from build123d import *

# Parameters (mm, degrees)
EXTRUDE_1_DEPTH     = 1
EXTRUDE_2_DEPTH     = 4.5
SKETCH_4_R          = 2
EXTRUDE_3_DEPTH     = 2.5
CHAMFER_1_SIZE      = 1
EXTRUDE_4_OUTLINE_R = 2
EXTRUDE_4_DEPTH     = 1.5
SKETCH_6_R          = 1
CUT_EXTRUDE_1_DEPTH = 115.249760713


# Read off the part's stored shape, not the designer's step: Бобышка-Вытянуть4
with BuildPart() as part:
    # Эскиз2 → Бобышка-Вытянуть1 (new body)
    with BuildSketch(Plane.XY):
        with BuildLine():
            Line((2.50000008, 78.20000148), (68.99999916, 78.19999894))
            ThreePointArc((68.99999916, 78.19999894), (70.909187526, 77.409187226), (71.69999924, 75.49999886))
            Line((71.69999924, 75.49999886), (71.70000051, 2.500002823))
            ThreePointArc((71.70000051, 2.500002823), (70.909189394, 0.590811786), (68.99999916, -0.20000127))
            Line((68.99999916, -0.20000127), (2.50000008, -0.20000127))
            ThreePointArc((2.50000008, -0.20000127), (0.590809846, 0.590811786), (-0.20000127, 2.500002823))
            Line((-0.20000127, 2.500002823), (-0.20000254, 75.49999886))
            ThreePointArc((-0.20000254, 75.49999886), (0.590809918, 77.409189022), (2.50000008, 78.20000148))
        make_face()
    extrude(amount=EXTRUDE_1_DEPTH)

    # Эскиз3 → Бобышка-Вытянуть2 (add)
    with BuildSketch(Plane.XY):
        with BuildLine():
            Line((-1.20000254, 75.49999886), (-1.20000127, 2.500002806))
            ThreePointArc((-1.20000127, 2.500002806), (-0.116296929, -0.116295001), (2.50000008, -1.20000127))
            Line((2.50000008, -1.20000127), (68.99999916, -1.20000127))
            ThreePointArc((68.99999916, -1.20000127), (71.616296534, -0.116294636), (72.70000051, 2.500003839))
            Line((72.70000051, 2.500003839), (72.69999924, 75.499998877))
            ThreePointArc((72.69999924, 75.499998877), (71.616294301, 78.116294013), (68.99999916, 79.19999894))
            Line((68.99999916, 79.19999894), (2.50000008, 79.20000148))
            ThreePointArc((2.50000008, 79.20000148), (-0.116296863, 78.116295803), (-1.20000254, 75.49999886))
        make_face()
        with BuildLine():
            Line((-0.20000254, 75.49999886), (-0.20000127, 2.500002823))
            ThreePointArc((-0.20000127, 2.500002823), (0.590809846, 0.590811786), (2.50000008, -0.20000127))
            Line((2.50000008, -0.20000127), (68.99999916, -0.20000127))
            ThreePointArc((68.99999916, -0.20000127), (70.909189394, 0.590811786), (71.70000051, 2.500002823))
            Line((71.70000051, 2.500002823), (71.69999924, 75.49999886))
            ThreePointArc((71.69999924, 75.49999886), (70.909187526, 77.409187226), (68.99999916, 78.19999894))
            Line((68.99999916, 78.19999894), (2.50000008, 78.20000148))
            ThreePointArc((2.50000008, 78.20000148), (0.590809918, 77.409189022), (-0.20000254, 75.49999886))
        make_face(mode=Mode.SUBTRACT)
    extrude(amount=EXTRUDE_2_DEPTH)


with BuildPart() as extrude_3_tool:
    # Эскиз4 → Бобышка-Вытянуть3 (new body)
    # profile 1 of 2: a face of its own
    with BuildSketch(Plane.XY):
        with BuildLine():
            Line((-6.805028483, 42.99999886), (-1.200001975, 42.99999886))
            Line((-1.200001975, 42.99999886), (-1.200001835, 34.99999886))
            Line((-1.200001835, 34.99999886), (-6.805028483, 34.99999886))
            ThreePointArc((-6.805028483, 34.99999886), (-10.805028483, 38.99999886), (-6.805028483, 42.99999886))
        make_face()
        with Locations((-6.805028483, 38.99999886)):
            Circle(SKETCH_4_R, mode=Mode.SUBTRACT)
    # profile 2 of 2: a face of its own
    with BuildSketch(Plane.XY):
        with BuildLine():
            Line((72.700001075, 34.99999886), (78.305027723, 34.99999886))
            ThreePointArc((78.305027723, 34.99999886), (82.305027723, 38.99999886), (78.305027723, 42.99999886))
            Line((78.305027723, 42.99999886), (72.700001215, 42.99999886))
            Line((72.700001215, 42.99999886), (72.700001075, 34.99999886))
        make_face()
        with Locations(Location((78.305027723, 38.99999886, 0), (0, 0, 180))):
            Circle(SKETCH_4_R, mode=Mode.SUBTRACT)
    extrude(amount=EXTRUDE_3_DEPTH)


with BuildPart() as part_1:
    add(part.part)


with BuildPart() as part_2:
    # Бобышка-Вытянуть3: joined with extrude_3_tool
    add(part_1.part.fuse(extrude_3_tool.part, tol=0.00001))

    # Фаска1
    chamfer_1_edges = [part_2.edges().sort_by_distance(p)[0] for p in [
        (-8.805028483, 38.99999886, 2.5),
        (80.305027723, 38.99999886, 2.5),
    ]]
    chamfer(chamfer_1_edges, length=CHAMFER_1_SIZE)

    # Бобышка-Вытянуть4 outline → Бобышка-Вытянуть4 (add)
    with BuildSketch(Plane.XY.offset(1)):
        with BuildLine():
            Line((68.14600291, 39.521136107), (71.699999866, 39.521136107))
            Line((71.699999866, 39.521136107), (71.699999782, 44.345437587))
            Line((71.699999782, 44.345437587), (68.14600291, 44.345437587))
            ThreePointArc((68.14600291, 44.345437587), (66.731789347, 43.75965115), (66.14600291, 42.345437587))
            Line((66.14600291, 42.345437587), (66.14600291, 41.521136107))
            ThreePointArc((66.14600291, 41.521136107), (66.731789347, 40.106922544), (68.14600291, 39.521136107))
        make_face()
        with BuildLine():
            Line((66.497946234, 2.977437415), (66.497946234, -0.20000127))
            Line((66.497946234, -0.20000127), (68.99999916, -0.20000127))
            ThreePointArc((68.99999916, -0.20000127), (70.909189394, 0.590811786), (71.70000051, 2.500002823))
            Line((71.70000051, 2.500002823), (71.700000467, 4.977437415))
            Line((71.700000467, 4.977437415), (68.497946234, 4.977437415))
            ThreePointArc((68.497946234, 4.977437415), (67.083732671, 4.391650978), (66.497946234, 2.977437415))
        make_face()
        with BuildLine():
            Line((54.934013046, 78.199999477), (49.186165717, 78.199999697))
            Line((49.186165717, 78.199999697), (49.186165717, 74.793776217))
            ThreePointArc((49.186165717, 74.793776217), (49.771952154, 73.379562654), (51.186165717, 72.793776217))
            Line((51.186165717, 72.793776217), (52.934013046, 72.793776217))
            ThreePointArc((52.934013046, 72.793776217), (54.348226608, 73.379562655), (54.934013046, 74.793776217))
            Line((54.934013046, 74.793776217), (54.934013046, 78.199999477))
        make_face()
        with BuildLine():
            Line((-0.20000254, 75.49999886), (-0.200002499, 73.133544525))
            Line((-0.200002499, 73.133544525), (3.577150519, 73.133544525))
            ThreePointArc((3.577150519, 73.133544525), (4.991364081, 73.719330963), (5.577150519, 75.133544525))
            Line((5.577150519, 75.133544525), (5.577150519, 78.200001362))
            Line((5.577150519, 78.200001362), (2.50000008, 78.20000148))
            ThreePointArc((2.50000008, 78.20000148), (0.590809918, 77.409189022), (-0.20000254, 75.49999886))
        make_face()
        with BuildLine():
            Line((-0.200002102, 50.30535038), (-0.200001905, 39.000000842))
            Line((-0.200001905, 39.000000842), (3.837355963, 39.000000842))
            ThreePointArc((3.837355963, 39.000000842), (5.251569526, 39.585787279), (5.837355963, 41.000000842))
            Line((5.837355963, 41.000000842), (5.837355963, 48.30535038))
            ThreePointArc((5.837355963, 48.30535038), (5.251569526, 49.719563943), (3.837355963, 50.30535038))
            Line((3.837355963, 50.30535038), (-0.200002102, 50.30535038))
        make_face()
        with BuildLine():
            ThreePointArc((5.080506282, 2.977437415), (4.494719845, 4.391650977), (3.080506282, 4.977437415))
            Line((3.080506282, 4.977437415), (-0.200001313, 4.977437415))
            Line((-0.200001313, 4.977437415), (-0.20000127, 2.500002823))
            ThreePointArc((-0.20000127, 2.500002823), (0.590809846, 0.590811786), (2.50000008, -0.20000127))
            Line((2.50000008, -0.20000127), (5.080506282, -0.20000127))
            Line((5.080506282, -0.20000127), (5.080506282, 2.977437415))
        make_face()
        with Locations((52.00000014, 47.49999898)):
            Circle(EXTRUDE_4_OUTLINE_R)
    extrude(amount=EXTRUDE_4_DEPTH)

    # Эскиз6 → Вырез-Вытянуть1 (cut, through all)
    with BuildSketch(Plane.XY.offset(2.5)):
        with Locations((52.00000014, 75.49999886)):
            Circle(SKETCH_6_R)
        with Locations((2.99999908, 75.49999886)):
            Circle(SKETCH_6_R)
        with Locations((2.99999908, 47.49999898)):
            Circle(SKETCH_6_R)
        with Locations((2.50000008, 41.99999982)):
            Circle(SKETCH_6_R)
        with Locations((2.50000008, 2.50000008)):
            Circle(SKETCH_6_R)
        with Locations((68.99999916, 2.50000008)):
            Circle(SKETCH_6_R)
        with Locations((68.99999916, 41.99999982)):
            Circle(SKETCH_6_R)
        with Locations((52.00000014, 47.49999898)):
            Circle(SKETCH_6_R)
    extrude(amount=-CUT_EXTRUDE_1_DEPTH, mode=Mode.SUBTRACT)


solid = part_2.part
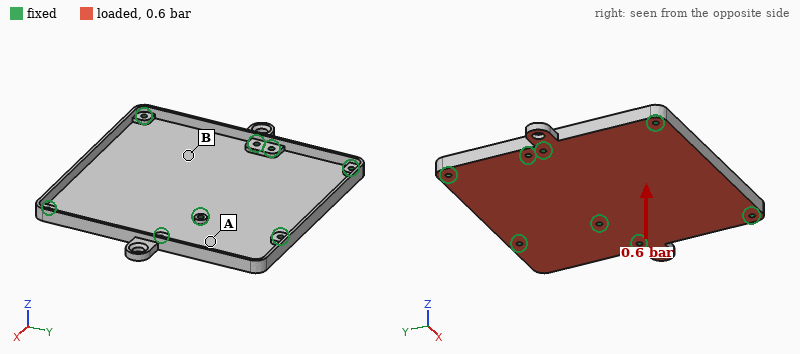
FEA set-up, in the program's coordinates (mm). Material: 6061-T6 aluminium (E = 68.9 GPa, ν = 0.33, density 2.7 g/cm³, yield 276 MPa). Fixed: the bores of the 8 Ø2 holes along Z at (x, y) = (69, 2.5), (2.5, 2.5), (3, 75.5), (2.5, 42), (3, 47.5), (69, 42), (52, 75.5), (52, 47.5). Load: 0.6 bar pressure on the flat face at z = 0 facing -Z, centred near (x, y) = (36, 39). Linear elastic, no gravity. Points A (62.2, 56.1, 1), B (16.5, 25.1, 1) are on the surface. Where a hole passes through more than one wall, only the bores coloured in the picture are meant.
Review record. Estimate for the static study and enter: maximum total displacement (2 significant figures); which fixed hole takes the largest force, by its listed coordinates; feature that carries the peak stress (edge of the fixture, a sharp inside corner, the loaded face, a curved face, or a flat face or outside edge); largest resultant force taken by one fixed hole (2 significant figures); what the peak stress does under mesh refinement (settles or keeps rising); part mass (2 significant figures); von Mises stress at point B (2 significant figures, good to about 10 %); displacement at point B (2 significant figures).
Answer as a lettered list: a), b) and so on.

a) 0.27 mm
b) (52, 47.5)
c) edge of the fixture
d) 84 N
e) keeps rising
f) 20 g
g) 24 MPa
h) 0.17 mm
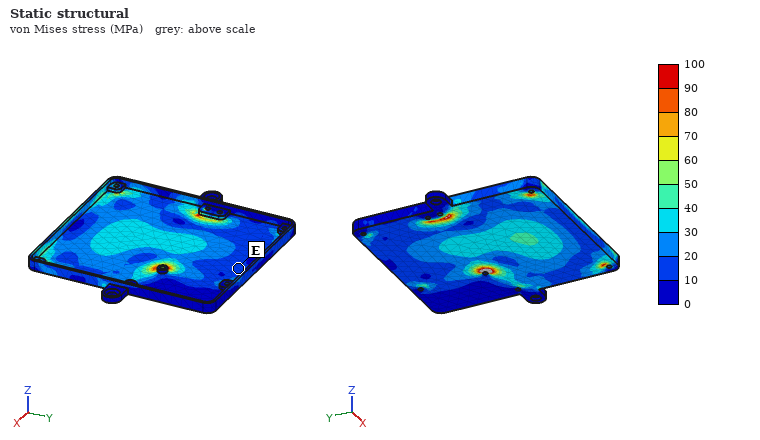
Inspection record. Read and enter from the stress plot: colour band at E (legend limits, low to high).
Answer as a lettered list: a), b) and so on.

a) 10 to 20 MPa
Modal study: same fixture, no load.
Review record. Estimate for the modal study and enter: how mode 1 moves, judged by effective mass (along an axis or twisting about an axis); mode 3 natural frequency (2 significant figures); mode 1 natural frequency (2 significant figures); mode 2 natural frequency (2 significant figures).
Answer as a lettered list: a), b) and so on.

a) along Z
b) 3600 Hz
c) 1800 Hz
d) 2800 Hz
